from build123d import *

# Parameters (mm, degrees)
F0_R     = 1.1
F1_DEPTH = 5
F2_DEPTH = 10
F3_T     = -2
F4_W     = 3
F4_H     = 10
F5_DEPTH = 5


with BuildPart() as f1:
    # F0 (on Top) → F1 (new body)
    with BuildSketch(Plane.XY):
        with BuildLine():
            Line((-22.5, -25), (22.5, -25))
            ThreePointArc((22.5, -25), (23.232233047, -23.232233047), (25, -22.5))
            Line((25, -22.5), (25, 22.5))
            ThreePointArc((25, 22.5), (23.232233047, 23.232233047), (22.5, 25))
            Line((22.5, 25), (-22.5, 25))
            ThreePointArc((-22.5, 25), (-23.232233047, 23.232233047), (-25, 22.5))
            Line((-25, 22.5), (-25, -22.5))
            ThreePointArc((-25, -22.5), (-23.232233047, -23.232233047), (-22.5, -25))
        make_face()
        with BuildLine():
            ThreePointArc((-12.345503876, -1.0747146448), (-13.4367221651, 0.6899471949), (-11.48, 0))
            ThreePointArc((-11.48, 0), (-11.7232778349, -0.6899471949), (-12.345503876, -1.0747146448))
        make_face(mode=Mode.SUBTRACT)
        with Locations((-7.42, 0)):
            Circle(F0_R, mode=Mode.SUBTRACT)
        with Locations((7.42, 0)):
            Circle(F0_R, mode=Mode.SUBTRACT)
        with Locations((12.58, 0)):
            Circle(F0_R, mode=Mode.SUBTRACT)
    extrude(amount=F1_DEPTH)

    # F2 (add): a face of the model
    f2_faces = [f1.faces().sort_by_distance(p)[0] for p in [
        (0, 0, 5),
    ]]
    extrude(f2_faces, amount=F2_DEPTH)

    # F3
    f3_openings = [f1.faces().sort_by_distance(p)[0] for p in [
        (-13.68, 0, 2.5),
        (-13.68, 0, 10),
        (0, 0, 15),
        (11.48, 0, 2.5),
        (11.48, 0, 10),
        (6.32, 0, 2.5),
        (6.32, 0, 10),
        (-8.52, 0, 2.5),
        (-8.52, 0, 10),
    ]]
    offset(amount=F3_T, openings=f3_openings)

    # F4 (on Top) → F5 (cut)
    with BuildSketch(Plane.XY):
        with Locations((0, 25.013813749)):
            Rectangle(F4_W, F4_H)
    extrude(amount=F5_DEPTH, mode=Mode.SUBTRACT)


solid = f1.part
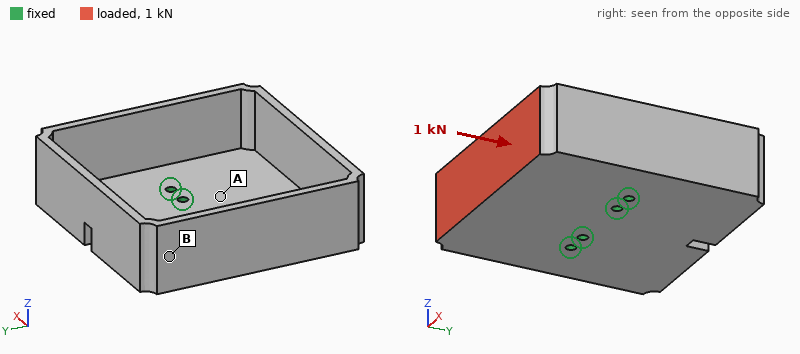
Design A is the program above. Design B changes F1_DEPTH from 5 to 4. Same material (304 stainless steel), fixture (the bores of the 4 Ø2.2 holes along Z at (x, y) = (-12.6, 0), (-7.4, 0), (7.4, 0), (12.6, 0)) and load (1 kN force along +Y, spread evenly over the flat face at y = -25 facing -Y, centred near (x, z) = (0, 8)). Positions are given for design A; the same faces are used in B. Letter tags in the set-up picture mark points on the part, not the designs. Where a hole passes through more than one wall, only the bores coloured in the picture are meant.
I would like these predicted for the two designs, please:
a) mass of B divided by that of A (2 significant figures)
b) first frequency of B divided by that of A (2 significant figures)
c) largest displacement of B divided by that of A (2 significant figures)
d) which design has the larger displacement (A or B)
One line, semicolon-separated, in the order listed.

0.96; 1.0; 0.92; A
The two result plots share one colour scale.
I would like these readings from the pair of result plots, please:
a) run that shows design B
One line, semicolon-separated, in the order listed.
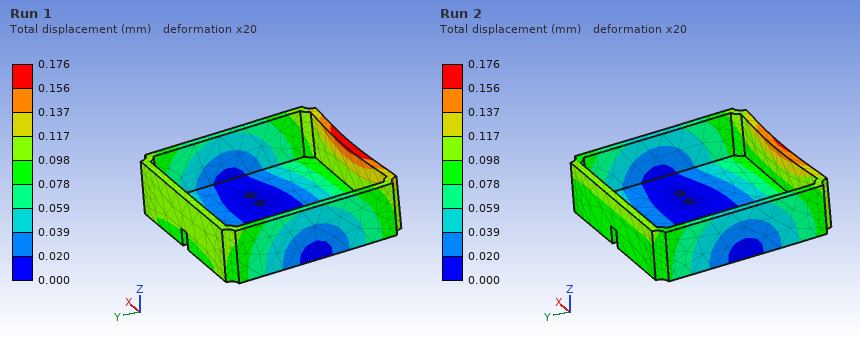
Run 2
